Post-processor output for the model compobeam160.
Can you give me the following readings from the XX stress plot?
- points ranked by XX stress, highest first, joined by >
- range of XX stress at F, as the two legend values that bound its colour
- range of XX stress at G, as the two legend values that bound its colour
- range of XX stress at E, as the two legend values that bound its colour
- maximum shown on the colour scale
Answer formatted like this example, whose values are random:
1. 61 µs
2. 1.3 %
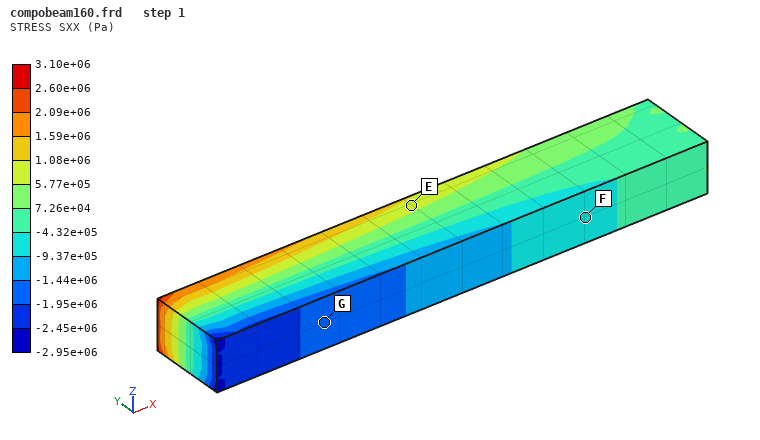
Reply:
1. E > F > G
2. -9.37e+05 to -4.32e+05 Pa
3. -1.95e+06 to -1.44e+06 Pa
4. 5.77e+05 to 1.08e+06 Pa
5. 3.10e+06 Pa
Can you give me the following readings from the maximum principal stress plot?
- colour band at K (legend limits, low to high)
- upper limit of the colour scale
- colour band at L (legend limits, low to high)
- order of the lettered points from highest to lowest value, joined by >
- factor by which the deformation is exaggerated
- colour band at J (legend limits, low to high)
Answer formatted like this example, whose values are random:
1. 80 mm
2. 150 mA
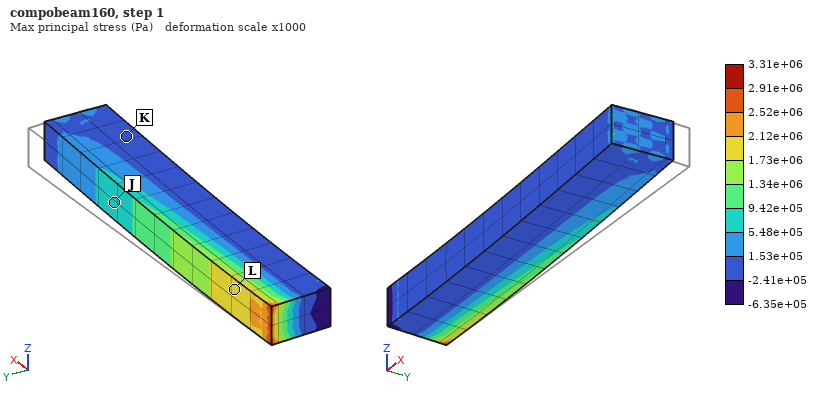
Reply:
1. -2.41e+05 to 1.53e+05 Pa
2. 3.31e+06 Pa
3. 1.73e+06 to 2.12e+06 Pa
4. L > J > K
5. 1000
6. 5.48e+05 to 9.42e+05 Pa
